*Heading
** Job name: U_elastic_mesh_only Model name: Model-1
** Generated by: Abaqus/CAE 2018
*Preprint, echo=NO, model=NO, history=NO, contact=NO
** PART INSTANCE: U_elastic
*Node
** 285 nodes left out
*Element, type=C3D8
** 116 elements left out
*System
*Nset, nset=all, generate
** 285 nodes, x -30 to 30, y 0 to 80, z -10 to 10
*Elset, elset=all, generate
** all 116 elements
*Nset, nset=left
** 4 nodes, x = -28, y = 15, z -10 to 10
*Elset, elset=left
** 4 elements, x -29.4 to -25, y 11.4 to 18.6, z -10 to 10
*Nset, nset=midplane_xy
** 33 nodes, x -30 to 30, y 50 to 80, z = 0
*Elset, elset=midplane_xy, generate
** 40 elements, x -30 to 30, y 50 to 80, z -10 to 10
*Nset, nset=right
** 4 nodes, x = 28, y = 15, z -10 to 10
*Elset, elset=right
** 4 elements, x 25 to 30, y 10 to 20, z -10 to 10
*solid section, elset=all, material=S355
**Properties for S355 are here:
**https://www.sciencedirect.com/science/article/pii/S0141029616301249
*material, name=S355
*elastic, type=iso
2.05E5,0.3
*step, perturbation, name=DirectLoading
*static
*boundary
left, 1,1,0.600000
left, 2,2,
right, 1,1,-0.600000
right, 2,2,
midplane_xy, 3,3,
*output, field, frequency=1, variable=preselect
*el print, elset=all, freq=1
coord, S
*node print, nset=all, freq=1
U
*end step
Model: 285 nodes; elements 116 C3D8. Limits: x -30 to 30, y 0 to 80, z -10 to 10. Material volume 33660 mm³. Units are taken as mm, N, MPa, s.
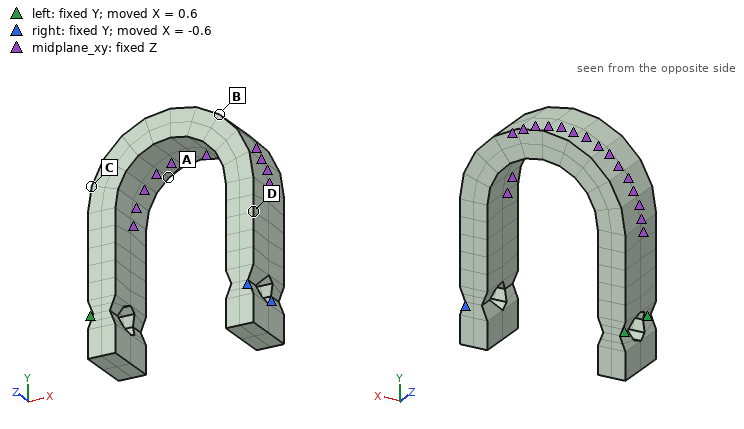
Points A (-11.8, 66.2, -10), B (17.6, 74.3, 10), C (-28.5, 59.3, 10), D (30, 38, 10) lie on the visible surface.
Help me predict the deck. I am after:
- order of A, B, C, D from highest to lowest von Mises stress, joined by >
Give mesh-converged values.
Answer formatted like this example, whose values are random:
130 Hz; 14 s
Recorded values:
A > B > C > D
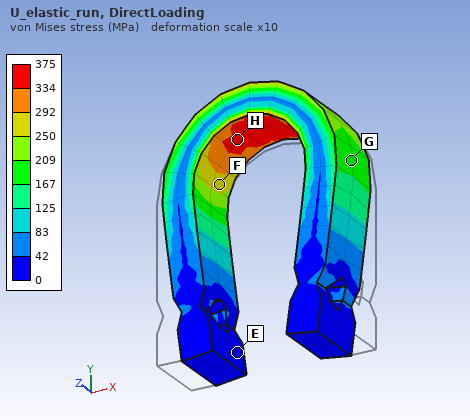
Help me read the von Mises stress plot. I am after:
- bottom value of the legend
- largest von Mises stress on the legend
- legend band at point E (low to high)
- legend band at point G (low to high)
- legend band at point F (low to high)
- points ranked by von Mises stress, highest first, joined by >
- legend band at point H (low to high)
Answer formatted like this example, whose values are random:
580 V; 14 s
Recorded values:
0 MPa; 375 MPa; 0 to 42 MPa; 167 to 209 MPa; 250 to 292 MPa; H > F > G > E; 334 to 375 MPa
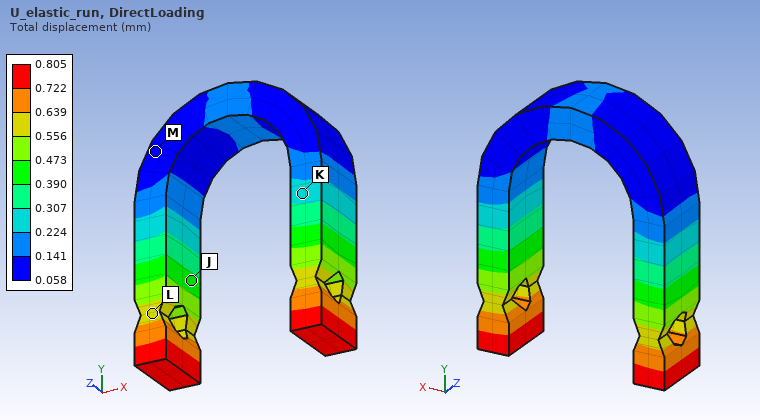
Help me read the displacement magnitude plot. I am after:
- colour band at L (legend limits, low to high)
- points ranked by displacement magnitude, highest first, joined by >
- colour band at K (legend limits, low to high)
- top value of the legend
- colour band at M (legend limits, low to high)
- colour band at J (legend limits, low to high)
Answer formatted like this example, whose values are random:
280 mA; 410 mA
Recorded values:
0.556 to 0.639 mm; L > J > K > M; 0.224 to 0.307 mm; 0.805 mm; 0.058 to 0.141 mm; 0.390 to 0.473 mm
